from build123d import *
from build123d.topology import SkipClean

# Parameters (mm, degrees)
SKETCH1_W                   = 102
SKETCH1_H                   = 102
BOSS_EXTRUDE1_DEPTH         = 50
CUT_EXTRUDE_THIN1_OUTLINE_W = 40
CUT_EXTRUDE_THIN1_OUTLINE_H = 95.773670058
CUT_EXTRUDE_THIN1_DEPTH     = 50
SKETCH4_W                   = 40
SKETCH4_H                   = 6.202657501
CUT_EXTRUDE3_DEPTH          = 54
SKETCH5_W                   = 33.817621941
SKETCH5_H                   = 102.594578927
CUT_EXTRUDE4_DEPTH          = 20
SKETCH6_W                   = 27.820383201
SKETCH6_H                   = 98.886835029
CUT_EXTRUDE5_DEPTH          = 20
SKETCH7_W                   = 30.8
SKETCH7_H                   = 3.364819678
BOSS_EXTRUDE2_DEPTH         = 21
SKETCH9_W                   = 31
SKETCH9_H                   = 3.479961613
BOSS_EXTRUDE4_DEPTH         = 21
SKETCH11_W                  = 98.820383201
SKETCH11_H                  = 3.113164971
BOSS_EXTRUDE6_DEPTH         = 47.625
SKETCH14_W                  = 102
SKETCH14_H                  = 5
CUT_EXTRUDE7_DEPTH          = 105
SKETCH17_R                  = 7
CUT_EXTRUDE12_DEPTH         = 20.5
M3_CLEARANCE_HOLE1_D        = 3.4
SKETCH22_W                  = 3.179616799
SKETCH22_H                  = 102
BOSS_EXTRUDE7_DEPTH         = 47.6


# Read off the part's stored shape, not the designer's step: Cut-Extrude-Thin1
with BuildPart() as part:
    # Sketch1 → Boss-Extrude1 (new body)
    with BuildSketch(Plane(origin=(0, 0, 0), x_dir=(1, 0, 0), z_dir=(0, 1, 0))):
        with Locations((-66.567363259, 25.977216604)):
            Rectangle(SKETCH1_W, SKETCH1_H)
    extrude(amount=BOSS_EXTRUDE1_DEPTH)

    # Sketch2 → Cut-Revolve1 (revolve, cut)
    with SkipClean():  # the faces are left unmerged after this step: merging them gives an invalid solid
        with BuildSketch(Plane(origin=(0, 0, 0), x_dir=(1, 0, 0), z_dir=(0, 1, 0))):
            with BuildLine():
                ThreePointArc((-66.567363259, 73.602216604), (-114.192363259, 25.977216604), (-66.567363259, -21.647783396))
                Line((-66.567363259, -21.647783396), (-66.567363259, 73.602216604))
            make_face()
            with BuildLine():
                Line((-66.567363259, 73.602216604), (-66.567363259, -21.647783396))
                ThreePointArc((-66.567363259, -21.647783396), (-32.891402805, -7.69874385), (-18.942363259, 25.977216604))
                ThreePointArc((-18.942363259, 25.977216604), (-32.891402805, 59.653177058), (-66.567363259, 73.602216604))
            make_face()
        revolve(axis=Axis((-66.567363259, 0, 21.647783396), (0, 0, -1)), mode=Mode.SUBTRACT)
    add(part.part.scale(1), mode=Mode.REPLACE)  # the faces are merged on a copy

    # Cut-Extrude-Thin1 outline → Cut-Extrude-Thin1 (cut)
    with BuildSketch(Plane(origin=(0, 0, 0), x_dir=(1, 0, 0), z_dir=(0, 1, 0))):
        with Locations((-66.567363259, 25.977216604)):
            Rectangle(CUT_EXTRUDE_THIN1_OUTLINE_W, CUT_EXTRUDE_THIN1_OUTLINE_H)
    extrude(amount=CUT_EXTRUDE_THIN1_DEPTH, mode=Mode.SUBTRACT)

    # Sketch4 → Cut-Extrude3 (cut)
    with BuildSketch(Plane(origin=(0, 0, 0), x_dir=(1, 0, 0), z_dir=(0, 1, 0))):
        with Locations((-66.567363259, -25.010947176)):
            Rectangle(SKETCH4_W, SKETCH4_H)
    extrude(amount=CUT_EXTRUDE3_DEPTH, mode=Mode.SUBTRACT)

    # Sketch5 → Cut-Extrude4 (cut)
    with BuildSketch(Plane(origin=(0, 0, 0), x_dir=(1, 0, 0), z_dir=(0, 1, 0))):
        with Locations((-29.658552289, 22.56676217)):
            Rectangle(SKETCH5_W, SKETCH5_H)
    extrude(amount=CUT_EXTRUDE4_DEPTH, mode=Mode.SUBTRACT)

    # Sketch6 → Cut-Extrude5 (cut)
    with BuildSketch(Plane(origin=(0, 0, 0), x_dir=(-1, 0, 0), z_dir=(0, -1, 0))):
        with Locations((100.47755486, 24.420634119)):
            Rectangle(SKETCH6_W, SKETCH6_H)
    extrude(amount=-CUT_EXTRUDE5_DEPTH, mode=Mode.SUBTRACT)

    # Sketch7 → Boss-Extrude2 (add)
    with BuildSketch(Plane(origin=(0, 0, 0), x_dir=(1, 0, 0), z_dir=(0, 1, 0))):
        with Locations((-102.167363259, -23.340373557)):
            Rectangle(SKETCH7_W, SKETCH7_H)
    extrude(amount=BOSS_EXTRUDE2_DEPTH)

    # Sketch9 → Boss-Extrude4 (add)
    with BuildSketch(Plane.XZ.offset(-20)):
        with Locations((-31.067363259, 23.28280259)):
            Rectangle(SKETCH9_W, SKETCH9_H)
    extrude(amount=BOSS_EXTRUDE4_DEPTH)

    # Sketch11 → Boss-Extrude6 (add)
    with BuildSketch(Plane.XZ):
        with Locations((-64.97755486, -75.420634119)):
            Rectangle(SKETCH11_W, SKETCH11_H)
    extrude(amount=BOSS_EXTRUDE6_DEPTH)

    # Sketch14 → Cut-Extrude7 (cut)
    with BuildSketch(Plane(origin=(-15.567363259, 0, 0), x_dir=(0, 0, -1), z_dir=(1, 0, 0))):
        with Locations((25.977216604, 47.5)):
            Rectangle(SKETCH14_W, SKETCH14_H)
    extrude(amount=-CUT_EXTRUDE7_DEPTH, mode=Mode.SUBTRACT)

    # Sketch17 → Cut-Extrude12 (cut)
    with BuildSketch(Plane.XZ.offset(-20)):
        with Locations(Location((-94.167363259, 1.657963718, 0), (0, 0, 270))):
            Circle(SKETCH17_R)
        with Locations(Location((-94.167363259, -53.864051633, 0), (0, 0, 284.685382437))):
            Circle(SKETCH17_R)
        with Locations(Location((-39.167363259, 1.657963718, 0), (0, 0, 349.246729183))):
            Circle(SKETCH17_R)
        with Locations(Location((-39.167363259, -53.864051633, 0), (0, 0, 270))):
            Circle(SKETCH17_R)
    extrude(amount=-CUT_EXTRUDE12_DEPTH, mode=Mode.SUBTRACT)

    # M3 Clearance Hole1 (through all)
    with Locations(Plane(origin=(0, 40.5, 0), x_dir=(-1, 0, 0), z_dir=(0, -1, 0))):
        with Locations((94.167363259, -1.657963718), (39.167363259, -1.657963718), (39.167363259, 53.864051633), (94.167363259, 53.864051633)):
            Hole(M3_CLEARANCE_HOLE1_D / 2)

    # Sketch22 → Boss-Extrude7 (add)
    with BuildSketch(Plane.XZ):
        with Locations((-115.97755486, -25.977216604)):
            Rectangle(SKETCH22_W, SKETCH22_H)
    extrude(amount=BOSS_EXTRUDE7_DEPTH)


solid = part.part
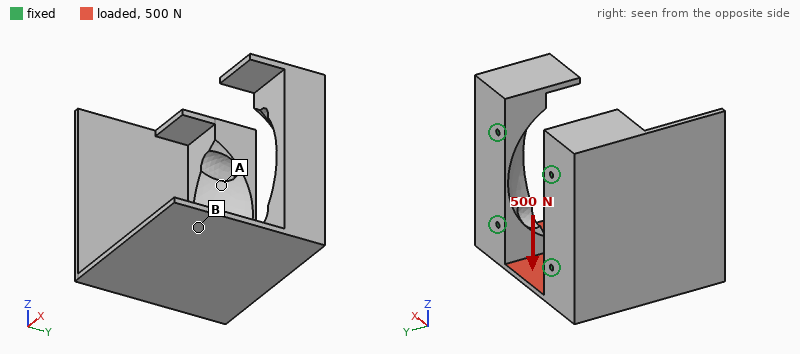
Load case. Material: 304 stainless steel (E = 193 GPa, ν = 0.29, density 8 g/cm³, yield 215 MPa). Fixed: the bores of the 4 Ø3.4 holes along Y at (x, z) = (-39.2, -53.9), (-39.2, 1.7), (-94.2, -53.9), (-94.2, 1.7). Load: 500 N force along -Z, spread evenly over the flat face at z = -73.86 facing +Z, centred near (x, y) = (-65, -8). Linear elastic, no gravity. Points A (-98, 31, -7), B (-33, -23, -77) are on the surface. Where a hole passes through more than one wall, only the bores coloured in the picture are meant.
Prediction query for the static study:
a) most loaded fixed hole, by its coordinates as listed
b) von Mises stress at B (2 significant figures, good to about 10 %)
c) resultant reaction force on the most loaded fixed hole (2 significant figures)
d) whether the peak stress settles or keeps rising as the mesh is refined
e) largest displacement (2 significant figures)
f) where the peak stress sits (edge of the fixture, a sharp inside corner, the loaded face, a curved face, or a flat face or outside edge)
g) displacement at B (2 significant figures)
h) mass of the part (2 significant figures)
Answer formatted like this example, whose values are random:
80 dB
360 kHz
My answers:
(-94.2, -53.9)
13 MPa
370 N
keeps rising
0.26 mm
edge of the fixture
0.14 mm
1.4 kg
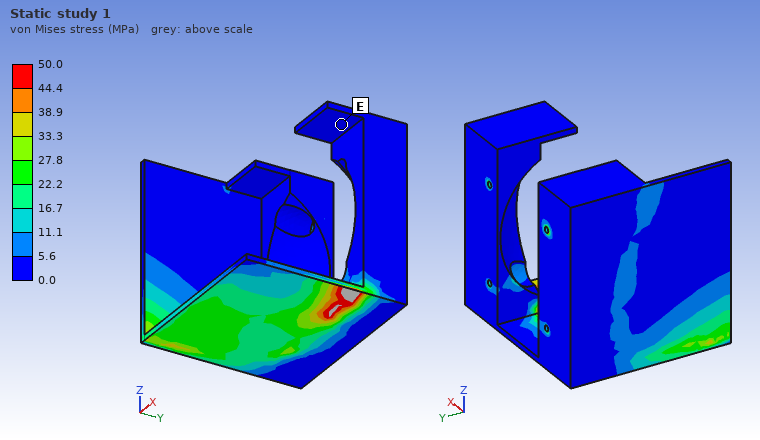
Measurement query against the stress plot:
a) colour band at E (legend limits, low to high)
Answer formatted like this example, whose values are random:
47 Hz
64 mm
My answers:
0.0 to 5.6 MPa
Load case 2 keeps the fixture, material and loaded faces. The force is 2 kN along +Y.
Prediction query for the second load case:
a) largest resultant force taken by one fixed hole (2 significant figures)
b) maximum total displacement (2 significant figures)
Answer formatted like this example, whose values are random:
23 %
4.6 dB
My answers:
1.5 kN
42 µm
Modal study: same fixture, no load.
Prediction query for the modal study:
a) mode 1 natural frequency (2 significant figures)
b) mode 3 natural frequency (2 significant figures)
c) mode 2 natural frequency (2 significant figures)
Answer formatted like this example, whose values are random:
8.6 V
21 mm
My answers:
680 Hz
1700 Hz
870 Hz
